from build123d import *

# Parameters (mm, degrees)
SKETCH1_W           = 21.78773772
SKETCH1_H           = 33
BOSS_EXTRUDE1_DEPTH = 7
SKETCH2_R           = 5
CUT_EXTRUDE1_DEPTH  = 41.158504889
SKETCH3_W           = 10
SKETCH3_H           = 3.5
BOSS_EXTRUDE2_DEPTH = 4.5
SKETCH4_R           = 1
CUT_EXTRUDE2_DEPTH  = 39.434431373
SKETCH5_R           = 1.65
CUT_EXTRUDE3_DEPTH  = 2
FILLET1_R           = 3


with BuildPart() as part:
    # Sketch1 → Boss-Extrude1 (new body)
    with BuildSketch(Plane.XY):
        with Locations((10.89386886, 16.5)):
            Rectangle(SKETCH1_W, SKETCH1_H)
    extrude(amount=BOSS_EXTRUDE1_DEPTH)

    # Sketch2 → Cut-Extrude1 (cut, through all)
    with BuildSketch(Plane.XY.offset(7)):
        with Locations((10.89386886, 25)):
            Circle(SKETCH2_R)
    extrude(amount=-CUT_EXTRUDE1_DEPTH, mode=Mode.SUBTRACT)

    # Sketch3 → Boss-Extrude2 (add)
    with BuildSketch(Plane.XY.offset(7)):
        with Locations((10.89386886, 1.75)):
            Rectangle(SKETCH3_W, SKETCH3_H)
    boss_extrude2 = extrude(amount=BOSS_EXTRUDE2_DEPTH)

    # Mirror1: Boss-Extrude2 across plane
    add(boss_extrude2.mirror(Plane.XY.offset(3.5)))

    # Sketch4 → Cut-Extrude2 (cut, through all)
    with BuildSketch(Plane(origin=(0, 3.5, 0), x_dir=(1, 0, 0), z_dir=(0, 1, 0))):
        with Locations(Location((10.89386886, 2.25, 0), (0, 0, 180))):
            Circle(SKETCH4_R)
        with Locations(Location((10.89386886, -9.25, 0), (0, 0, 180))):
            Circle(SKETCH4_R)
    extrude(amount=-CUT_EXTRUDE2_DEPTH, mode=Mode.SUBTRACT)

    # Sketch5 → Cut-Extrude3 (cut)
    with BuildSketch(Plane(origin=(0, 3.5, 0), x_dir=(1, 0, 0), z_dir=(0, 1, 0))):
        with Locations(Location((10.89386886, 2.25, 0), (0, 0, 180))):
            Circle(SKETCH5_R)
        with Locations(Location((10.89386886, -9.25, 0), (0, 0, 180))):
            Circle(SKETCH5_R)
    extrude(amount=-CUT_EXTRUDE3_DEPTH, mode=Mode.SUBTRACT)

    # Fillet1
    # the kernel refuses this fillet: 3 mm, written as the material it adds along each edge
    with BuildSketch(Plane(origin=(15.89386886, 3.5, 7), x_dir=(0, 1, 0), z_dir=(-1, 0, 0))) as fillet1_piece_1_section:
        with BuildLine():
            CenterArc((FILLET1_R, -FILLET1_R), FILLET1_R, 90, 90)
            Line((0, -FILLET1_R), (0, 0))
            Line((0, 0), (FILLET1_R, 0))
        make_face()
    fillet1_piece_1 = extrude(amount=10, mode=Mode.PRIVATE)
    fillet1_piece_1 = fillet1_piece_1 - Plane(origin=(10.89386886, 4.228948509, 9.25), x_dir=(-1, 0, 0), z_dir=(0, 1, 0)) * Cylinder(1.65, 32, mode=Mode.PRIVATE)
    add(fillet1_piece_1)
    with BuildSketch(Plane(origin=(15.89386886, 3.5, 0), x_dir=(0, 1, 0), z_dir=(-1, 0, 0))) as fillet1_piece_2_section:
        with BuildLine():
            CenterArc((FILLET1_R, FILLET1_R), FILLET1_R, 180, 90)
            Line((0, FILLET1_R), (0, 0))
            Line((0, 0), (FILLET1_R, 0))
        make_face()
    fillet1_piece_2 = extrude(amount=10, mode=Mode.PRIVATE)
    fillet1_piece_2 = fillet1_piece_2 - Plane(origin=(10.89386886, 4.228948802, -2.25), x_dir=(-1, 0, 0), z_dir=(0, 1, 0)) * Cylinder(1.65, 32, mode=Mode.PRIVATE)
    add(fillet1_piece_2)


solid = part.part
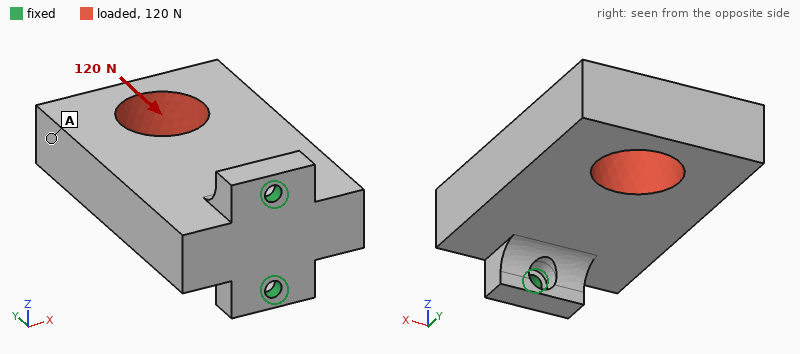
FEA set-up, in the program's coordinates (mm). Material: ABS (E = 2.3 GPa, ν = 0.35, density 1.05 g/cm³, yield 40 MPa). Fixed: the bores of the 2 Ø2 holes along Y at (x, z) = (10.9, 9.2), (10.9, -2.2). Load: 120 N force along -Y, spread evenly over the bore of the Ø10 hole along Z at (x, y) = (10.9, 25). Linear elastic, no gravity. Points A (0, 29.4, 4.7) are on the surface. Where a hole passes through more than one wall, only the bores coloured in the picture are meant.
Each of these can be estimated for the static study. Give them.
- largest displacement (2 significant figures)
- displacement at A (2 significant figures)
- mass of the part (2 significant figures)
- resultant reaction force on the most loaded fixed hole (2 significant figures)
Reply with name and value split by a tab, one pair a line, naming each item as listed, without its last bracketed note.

largest displacement	38 µm
displacement at A	26 µm
mass of the part	5.0 g
resultant reaction force on the most loaded fixed hole	65 N
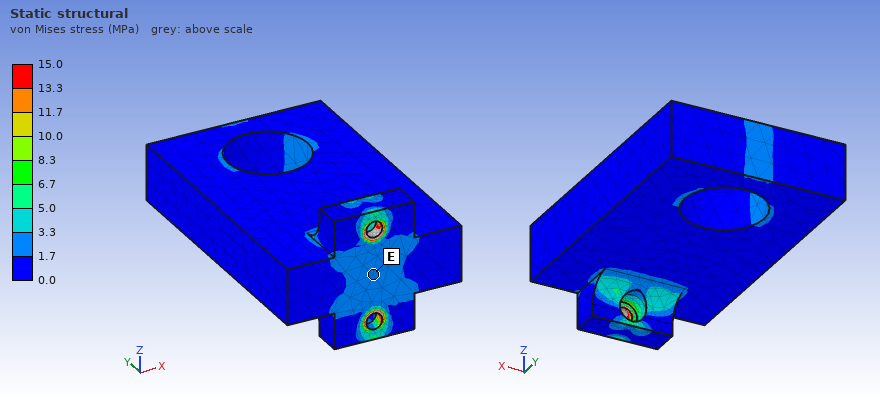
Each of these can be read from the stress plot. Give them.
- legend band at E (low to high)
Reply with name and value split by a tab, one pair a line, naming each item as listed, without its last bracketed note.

legend band at E	1.7 to 3.3 MPa
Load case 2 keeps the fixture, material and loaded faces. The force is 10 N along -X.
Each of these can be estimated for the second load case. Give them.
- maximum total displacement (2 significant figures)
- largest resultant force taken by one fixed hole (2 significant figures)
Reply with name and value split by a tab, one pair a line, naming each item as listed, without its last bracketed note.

maximum total displacement	0.45 mm
largest resultant force taken by one fixed hole	5.0 N
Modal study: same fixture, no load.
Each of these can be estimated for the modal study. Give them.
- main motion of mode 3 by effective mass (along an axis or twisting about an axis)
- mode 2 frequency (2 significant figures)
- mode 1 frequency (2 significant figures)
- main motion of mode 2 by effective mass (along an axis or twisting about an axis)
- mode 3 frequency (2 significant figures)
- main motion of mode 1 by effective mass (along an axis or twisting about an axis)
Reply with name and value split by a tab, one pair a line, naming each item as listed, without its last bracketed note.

main motion of mode 3 by effective mass	twisting about Y
mode 2 frequency	1400 Hz
mode 1 frequency	530 Hz
main motion of mode 2 by effective mass	along Z
mode 3 frequency	3500 Hz
main motion of mode 1 by effective mass	along X
